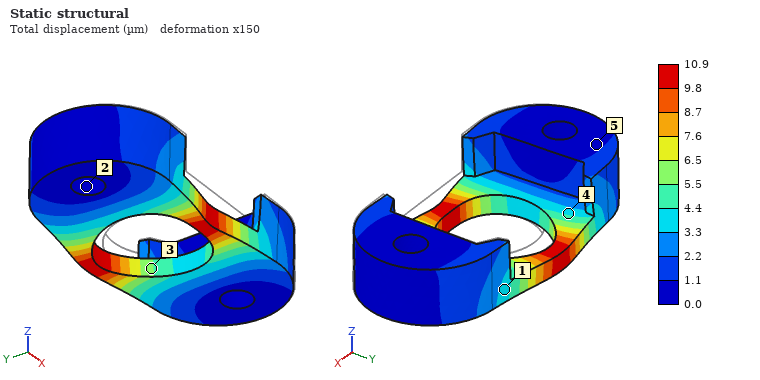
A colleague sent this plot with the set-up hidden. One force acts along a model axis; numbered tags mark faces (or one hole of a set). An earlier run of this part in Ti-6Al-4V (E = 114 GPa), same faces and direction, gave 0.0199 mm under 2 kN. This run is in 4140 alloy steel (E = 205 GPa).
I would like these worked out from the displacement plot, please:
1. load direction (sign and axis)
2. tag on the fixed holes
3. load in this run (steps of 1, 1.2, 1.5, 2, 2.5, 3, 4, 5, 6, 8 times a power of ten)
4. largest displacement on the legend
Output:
+Y
2
2 kN
10.9 µm
